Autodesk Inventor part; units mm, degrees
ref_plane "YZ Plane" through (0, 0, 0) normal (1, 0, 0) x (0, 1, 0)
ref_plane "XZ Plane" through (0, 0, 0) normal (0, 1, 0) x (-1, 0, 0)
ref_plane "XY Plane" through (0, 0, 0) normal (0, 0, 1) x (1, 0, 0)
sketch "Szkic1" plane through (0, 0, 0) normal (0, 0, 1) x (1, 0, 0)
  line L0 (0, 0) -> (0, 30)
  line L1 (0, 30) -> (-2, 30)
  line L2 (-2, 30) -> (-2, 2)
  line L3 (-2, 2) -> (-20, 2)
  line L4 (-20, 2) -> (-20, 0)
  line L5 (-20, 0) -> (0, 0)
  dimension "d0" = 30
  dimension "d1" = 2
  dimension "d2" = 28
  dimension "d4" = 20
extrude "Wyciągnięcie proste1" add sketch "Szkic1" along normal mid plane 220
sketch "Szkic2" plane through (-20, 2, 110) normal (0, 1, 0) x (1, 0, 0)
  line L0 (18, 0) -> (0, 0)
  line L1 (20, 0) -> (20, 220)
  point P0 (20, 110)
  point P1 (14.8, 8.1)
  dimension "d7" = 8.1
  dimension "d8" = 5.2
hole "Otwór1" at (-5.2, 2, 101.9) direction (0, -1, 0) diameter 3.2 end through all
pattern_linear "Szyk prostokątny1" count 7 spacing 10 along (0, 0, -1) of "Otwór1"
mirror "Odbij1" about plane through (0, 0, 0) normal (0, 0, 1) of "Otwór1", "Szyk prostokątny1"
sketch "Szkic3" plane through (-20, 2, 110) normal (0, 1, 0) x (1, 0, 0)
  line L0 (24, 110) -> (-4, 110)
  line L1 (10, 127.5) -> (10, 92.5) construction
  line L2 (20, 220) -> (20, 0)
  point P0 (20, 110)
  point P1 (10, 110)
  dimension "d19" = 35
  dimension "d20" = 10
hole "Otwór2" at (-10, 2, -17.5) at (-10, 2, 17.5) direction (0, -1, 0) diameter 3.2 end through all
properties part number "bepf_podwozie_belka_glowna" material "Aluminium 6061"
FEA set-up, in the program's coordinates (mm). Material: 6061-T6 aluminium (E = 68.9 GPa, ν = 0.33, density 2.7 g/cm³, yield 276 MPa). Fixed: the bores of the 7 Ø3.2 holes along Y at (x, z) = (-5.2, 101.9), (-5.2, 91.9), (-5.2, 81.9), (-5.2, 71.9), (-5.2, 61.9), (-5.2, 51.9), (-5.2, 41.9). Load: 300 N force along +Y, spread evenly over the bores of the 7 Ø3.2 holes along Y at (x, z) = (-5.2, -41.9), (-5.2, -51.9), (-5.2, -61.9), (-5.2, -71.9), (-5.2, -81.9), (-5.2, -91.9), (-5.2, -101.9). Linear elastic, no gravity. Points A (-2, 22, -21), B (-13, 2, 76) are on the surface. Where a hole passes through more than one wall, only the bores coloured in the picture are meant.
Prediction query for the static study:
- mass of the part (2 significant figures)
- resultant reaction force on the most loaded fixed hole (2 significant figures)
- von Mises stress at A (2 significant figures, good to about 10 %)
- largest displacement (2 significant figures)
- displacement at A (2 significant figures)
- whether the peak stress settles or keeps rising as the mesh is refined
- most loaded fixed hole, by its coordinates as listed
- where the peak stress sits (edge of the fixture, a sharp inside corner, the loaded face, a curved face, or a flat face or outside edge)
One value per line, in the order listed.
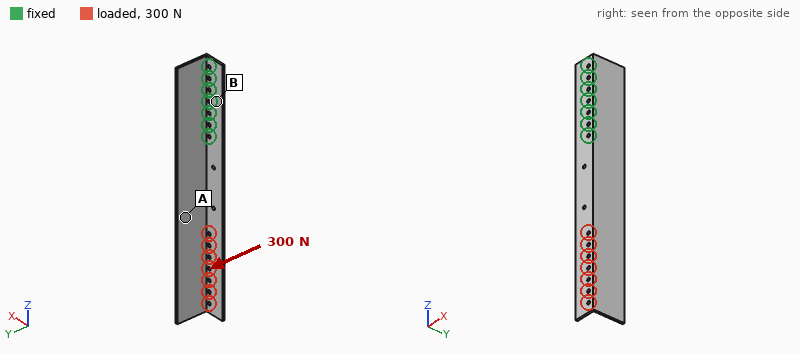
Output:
56 g
1.4 kN
48 MPa
1.8 mm
0.40 mm
keeps rising
(-5.2, 41.9)
edge of the fixture
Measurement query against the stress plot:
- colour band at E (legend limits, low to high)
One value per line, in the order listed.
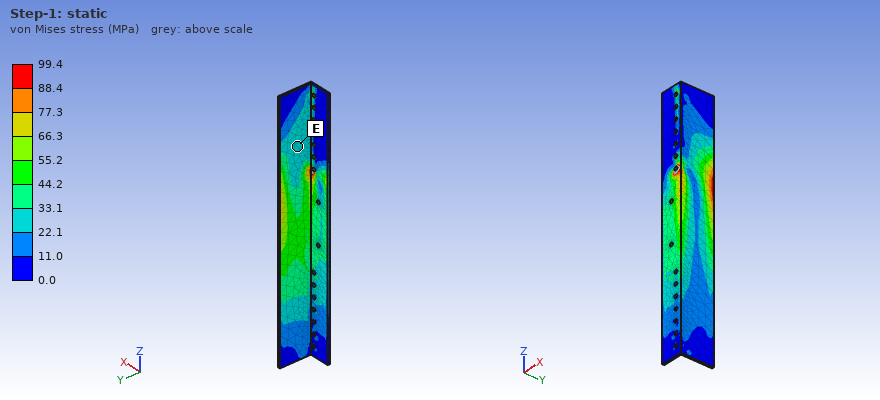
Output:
22.1 to 33.1 MPa
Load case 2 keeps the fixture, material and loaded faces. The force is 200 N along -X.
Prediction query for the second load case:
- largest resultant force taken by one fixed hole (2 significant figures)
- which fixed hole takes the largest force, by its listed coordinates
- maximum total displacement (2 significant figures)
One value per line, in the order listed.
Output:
1.2 kN
(-5.2, 41.9)
1.4 mm
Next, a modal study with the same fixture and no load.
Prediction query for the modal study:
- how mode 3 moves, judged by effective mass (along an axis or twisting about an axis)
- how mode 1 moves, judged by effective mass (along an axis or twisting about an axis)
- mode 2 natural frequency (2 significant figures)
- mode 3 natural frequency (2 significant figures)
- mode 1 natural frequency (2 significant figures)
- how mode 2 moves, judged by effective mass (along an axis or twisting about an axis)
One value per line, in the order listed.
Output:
along Y
along X
560 Hz
980 Hz
350 Hz
along Y
